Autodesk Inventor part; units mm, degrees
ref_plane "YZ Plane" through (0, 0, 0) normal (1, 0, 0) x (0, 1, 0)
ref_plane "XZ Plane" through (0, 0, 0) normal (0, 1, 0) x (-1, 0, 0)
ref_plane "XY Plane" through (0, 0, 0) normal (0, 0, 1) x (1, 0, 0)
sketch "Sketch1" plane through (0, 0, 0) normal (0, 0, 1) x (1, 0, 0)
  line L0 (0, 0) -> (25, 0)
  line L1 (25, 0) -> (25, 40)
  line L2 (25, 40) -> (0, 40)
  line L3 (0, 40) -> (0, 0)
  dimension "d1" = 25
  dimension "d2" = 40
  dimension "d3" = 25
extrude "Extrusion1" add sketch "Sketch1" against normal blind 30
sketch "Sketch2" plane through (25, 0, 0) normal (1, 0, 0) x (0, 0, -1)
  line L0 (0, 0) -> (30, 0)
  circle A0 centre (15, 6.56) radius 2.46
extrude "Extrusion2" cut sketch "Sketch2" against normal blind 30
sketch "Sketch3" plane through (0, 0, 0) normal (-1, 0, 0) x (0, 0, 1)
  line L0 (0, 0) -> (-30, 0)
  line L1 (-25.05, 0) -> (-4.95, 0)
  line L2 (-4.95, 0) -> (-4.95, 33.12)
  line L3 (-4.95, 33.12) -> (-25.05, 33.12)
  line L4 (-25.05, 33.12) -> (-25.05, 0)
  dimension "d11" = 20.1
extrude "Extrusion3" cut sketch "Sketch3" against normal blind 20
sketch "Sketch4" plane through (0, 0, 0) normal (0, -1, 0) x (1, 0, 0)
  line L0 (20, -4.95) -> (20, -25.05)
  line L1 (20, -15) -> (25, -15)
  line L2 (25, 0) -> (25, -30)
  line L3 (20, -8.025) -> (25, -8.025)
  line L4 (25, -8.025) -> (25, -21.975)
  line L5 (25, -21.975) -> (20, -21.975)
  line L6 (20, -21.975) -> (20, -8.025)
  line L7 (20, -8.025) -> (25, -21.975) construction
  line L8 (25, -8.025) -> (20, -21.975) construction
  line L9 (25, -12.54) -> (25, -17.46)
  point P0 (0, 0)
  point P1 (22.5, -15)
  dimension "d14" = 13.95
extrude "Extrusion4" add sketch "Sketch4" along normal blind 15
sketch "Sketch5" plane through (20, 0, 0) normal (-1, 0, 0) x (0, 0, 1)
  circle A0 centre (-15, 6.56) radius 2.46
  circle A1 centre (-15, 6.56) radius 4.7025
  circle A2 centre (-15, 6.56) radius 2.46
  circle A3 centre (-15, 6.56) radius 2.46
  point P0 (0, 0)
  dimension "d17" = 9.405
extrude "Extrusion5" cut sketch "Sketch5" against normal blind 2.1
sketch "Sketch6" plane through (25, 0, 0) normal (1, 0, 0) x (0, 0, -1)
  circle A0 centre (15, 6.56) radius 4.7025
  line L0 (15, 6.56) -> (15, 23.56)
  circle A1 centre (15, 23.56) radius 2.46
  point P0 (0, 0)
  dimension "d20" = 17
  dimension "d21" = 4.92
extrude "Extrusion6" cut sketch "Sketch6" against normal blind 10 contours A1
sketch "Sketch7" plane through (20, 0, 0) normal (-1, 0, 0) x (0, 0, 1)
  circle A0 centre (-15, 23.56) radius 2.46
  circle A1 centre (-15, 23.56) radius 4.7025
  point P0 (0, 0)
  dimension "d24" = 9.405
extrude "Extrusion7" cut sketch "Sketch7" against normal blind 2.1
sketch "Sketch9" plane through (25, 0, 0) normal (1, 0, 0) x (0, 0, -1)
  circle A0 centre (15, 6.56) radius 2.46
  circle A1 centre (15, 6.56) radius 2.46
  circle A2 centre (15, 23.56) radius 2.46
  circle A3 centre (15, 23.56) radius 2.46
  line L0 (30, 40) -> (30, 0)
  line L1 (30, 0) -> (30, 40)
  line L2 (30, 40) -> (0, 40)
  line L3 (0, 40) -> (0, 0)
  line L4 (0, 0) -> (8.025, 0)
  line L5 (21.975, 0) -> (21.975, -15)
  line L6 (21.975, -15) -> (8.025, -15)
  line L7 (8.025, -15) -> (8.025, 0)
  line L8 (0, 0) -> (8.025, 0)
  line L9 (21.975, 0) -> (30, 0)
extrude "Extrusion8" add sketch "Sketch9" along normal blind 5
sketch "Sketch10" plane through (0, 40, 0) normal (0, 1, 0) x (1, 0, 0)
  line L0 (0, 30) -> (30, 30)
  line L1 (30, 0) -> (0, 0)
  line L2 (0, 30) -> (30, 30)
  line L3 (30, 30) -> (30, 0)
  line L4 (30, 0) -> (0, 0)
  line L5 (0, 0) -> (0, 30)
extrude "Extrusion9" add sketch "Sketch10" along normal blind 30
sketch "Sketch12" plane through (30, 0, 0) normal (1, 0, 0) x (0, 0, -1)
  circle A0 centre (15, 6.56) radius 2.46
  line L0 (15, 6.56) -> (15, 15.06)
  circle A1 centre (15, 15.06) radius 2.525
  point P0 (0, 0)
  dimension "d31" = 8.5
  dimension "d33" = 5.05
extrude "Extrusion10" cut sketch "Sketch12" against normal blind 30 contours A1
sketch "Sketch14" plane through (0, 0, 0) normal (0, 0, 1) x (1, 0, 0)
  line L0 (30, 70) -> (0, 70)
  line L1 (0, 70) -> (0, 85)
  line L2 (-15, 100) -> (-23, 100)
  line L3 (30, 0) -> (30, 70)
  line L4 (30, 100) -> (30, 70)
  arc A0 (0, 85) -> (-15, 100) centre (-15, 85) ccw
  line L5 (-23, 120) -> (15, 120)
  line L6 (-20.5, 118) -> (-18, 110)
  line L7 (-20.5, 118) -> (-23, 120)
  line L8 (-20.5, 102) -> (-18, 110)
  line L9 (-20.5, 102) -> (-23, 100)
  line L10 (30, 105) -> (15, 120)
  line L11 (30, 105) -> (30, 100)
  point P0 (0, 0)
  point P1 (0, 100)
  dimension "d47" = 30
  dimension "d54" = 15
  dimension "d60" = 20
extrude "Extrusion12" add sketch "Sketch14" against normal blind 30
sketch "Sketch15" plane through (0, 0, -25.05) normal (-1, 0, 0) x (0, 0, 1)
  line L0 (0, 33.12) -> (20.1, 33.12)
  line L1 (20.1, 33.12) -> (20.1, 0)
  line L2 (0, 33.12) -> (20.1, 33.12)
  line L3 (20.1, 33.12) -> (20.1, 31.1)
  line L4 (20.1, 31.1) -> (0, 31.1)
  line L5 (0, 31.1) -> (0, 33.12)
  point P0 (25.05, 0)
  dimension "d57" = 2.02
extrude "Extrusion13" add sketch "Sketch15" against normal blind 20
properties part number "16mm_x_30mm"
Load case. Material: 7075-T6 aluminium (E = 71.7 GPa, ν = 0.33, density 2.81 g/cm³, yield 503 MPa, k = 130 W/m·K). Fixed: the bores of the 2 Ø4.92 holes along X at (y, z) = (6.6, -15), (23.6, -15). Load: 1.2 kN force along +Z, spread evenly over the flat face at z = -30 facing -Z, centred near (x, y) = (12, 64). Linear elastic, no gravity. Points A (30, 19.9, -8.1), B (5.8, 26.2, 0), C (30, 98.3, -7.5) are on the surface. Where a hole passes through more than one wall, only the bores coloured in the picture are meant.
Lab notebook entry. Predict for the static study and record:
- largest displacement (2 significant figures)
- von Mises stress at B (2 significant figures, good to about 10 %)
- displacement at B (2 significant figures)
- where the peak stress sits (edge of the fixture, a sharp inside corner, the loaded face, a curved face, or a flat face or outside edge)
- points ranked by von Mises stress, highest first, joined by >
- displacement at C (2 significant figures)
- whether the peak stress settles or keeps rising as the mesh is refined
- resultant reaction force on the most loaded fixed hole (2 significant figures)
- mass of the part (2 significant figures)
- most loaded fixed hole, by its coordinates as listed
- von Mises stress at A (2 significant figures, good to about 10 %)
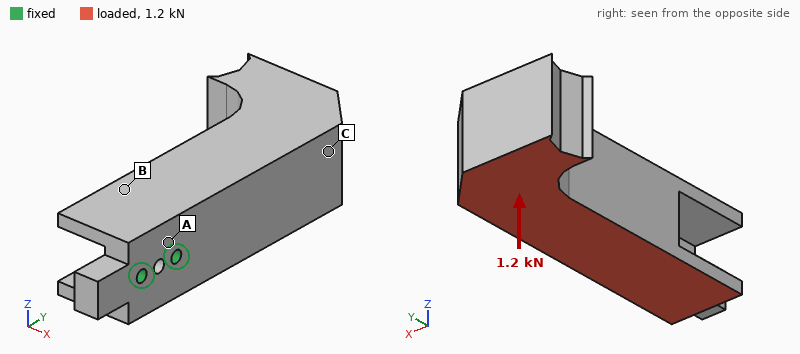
0.12 mm
9.4 MPa
0.018 mm
edge of the fixture
A > B > C
0.064 mm
keeps rising
3.2 kN
300 g
(23.6, -15)
19 MPa
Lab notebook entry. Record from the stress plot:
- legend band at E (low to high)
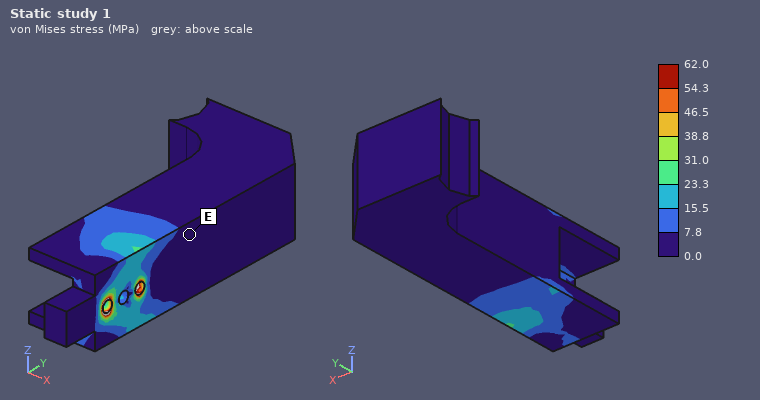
0.0 to 7.8 MPa
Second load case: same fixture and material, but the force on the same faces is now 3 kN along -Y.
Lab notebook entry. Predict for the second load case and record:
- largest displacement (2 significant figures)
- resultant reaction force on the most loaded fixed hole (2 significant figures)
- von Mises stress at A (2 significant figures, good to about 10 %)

0.13 mm
3.1 kN
22 MPa
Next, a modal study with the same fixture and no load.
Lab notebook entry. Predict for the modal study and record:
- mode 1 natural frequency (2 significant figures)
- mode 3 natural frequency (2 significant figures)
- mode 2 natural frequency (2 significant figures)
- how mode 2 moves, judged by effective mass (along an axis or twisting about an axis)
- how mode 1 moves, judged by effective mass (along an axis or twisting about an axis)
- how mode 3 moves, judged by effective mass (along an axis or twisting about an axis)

980 Hz
2900 Hz
1100 Hz
along Z
along X
twisting about Y
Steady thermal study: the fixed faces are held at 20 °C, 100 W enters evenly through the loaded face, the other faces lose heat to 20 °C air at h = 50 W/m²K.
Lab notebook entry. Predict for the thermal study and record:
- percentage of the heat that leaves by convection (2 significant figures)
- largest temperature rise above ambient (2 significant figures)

22 %
45 K
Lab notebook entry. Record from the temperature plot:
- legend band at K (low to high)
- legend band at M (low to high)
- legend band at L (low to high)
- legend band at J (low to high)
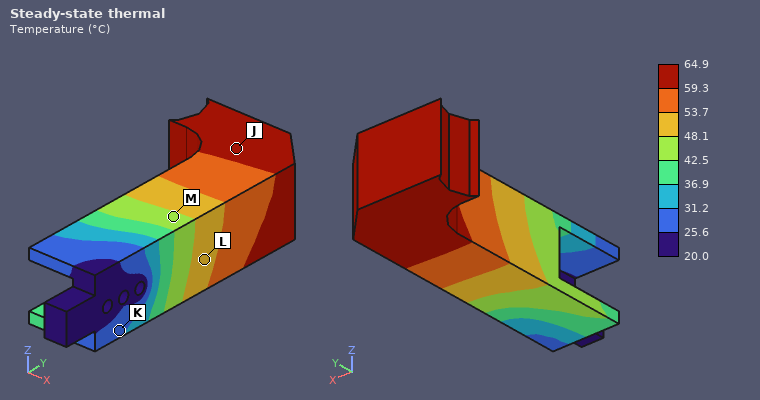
25.6 to 31.2 °C
42.5 to 48.1 °C
48.1 to 53.7 °C
59.3 to 64.9 °C
